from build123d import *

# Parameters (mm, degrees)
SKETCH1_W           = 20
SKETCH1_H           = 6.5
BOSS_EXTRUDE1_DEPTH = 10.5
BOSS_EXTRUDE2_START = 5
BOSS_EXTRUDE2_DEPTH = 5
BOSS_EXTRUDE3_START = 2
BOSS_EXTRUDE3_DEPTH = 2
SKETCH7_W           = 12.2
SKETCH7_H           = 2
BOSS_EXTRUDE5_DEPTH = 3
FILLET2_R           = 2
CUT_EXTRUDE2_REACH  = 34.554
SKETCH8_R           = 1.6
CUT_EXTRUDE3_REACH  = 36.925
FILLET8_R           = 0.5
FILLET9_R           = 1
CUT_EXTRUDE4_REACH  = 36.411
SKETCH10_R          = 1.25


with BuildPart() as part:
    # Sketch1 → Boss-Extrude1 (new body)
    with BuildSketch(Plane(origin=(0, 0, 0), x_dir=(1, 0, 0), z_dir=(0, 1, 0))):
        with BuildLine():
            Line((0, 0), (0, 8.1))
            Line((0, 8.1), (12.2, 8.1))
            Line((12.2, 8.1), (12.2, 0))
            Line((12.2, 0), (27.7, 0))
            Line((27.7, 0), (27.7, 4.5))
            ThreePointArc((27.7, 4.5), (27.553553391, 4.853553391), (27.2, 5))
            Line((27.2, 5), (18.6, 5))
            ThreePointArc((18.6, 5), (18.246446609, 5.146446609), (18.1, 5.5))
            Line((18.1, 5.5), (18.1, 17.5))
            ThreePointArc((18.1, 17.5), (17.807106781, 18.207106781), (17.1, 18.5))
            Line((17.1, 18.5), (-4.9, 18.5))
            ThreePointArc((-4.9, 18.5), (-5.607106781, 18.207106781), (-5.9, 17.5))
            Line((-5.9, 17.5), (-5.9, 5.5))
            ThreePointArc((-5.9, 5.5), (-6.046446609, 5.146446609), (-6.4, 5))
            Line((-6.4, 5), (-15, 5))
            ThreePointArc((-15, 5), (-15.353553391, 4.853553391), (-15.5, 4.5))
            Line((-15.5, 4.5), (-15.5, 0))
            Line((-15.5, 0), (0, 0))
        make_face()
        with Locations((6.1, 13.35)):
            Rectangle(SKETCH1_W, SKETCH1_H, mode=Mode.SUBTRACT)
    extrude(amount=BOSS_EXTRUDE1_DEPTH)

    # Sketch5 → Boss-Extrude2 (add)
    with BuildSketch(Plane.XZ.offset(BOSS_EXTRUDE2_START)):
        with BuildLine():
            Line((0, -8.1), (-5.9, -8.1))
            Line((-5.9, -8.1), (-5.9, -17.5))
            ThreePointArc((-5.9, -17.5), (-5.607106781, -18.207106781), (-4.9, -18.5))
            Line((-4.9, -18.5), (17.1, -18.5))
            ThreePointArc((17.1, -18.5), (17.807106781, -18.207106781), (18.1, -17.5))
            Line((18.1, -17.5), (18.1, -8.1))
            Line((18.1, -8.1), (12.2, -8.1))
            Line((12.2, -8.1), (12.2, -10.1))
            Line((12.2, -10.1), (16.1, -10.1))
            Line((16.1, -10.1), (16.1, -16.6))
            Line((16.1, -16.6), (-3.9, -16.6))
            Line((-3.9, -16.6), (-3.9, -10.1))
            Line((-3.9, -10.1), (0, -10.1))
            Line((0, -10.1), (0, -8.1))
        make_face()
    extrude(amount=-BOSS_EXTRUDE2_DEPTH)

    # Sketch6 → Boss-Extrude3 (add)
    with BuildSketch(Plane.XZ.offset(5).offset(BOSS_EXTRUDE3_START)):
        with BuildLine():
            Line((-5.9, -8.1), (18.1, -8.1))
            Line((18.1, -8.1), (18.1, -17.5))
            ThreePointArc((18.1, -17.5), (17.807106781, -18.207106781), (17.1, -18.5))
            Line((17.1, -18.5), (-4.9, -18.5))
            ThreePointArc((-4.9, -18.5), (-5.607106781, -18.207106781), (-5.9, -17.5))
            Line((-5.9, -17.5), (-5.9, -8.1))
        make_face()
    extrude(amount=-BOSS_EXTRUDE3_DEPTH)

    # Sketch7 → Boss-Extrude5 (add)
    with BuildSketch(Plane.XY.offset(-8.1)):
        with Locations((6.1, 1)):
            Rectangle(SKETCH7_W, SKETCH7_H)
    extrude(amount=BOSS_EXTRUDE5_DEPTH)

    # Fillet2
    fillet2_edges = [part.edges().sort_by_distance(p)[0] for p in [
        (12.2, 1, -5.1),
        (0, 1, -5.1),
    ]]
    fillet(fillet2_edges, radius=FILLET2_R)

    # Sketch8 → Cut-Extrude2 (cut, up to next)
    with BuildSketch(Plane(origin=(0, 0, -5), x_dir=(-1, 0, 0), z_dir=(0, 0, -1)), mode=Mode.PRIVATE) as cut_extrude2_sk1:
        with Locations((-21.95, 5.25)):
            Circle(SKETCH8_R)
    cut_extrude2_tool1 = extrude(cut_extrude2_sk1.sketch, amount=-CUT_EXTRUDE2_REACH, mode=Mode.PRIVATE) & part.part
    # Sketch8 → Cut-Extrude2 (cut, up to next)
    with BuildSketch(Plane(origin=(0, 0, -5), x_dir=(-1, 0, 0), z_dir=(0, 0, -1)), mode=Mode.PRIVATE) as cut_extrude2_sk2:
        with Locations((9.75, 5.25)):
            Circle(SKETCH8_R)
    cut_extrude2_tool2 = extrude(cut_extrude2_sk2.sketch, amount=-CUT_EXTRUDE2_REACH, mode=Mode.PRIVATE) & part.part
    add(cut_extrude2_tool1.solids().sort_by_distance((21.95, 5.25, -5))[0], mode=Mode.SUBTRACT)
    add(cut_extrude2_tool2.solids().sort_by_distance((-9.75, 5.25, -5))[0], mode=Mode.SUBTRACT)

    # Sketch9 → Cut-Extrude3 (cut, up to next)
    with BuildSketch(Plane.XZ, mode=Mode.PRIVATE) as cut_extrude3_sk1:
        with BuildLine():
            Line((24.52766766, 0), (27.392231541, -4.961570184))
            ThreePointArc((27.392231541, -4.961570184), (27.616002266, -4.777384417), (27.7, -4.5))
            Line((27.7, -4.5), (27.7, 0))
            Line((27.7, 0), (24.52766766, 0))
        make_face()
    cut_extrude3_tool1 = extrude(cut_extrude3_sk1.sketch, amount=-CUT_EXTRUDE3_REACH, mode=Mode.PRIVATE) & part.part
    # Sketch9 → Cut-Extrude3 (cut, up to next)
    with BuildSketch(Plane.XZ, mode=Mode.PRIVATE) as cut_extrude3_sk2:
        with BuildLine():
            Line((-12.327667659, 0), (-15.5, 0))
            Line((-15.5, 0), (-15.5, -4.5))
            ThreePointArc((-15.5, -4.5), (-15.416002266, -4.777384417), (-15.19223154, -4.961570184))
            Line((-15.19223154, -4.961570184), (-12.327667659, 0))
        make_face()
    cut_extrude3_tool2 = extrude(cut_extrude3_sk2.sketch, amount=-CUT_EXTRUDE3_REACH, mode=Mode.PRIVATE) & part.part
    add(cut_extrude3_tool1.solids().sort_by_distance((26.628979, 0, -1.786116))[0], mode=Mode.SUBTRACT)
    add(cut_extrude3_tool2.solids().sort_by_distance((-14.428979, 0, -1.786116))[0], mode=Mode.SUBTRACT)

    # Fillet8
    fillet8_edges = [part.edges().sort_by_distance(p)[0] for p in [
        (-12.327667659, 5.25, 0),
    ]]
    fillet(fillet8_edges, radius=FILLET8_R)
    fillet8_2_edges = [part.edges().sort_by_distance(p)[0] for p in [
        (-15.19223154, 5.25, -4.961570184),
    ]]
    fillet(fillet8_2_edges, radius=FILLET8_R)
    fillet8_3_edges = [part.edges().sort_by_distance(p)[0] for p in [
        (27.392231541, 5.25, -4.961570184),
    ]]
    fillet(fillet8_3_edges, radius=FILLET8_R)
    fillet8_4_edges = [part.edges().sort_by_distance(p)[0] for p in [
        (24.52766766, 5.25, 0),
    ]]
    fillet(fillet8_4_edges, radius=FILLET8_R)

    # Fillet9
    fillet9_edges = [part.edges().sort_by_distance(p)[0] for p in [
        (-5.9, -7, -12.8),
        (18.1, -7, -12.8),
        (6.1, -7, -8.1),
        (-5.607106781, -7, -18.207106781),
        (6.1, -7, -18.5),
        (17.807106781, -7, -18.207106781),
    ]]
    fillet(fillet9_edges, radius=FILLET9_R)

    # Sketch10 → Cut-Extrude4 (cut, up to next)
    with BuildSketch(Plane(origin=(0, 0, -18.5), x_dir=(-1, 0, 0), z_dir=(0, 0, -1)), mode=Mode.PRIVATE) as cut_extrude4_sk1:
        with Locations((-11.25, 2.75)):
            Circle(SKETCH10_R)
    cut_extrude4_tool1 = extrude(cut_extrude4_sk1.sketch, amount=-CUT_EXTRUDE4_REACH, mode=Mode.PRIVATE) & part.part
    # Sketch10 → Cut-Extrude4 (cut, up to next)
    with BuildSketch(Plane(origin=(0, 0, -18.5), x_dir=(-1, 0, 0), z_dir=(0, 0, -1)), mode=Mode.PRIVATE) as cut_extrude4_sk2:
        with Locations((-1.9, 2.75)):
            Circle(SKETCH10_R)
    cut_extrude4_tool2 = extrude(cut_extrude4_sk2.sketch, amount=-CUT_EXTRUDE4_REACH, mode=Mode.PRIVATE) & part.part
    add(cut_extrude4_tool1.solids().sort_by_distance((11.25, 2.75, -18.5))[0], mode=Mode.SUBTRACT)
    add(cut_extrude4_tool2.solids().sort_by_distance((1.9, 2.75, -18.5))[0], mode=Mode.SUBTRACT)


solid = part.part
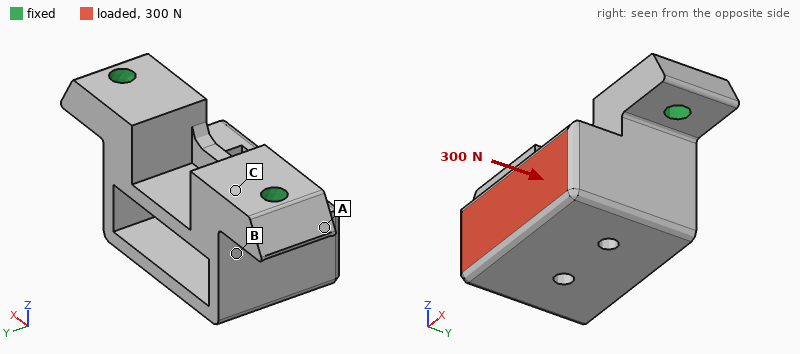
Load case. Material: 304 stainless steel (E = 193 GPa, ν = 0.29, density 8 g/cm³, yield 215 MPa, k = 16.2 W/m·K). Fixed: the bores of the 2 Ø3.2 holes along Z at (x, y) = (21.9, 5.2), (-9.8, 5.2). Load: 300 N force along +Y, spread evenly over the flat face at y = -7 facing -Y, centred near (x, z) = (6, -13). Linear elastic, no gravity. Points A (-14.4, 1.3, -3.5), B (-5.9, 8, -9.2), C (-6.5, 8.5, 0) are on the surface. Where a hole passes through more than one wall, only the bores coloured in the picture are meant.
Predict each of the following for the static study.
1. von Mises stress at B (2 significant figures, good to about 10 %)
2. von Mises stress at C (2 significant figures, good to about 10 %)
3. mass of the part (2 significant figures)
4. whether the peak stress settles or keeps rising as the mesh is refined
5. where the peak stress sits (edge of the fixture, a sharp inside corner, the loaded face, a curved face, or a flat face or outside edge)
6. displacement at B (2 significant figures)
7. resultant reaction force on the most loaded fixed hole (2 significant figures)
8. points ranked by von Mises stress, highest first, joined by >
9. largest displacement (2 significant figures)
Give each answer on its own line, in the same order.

10 MPa
17 MPa
32 g
keeps rising
edge of the fixture
2.9 µm
150 N
C > B > A
8.6 µm
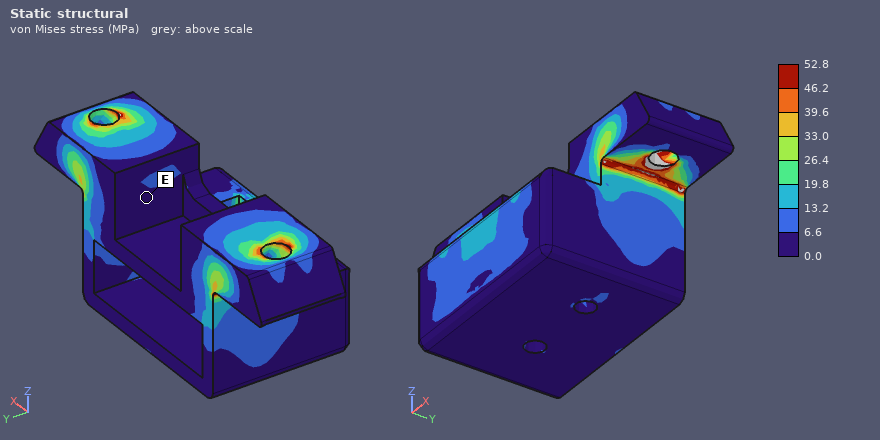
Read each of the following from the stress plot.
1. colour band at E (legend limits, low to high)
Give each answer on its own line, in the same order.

0.0 to 6.6 MPa
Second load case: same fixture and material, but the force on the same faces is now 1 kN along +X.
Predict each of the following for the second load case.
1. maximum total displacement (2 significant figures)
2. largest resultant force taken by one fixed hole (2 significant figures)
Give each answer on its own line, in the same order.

17 µm
710 N
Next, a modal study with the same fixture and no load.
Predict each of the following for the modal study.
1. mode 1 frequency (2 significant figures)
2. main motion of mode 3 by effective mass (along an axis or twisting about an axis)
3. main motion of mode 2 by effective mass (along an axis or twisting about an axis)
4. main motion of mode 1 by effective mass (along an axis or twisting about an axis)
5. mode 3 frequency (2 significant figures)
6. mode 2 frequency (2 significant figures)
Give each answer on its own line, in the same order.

7500 Hz
along X
along X
along Y
15 kHz
11 kHz
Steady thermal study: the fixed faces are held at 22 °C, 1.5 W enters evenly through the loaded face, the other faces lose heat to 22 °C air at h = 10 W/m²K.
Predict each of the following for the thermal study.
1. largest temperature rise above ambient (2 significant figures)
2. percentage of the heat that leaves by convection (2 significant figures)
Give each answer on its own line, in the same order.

24 K
21 %
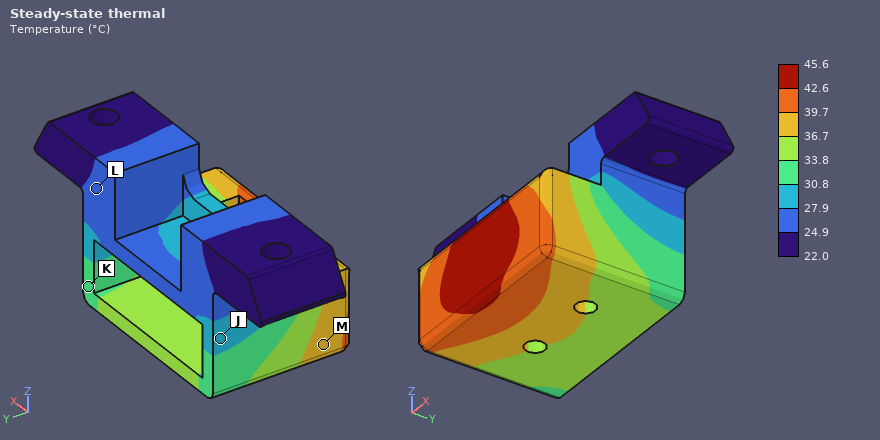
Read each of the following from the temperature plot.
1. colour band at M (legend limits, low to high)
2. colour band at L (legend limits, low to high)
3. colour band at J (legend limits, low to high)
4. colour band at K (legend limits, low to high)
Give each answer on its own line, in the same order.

36.7 to 39.7 °C
24.9 to 27.9 °C
27.9 to 30.8 °C
30.8 to 33.8 °C
